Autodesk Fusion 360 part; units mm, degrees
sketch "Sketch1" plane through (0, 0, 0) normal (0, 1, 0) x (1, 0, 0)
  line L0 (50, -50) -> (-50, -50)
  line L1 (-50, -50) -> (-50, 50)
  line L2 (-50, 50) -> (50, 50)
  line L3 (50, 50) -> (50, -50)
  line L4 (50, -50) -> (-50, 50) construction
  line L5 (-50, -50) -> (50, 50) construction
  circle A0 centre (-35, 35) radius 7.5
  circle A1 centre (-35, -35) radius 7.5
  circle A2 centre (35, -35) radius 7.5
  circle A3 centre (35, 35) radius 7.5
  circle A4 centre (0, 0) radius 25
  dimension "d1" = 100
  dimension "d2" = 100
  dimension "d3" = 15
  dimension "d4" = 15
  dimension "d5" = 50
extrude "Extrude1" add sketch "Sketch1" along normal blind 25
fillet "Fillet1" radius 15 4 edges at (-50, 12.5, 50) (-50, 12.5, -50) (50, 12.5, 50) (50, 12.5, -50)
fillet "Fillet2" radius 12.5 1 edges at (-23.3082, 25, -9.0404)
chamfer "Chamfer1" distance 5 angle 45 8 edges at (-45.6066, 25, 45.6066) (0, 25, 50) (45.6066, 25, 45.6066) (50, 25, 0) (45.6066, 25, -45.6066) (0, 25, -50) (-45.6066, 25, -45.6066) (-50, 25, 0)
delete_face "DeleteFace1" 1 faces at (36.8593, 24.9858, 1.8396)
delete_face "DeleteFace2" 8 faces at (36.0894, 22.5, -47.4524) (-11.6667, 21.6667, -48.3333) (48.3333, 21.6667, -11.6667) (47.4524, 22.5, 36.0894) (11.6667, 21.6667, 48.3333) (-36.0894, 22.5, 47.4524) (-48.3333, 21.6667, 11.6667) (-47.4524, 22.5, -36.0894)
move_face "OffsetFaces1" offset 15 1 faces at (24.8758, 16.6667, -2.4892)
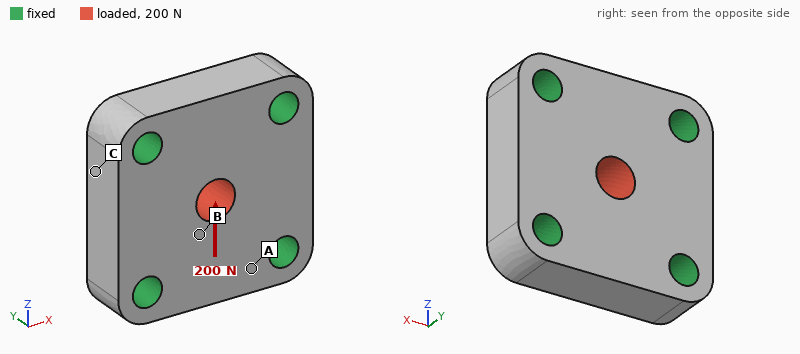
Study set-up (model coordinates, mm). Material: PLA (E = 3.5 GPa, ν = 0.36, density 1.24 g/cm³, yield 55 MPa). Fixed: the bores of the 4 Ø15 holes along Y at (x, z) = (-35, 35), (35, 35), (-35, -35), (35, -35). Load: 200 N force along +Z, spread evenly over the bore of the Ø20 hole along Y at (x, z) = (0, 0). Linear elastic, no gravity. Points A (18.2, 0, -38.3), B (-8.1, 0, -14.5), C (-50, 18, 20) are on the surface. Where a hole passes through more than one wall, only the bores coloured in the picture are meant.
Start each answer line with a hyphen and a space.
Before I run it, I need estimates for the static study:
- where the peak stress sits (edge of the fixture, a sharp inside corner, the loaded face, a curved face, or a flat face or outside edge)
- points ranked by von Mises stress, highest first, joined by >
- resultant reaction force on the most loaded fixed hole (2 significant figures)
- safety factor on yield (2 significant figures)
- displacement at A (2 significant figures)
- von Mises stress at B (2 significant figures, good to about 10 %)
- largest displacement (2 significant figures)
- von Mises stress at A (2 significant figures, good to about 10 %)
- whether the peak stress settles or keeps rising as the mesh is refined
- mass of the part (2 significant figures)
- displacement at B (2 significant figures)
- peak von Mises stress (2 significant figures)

- the loaded face
- B > A > C
- 56 N
- 250
- 0.45 µm
- 0.10 MPa
- 1.3 µm
- 0.061 MPa
- settles
- 270 g
- 0.97 µm
- 0.22 MPa
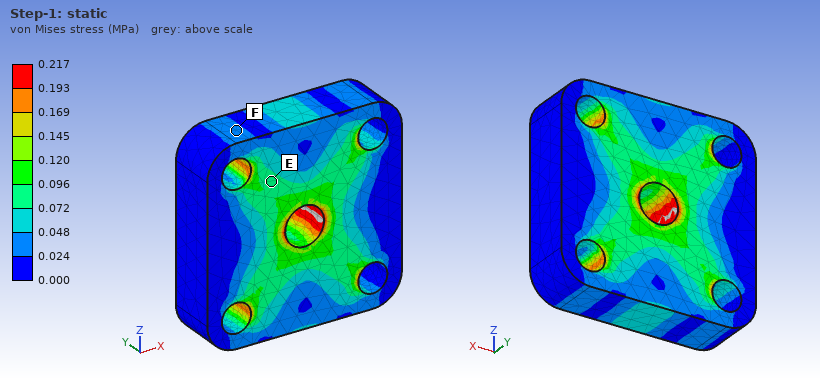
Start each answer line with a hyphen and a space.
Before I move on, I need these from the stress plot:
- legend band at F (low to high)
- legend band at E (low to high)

- 0.024 to 0.048 MPa
- 0.072 to 0.096 MPa
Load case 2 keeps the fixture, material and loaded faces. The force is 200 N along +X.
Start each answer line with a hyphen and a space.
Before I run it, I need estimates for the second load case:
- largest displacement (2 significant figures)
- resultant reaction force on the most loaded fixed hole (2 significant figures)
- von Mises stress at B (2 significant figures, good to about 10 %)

- 1.3 µm
- 56 N
- 0.095 MPa
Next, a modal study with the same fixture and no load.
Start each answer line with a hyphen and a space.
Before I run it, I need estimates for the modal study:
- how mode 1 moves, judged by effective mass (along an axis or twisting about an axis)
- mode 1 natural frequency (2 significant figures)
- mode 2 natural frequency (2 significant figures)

- along Y
- 4900 Hz
- 6600 Hz
